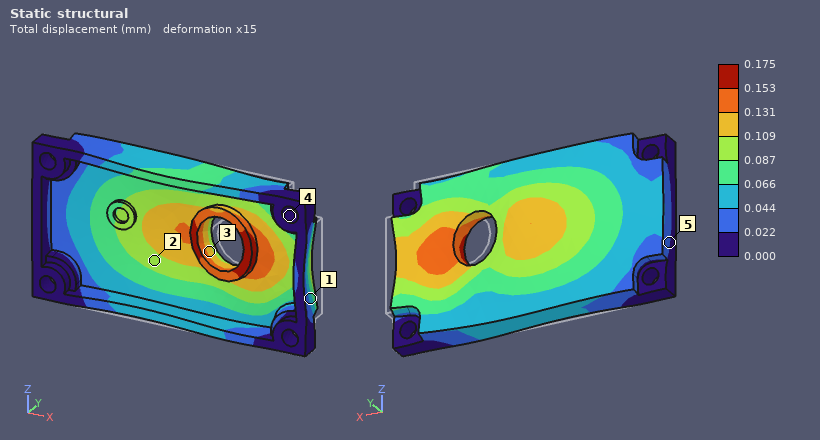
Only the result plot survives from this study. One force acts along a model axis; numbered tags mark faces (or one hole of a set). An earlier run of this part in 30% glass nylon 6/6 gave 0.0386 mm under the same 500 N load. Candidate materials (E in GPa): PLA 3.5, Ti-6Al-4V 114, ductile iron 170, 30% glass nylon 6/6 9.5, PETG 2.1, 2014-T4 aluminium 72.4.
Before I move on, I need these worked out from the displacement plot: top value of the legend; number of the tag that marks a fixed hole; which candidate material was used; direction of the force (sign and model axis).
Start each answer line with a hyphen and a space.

- 0.175 mm
- 4
- PETG
- -X
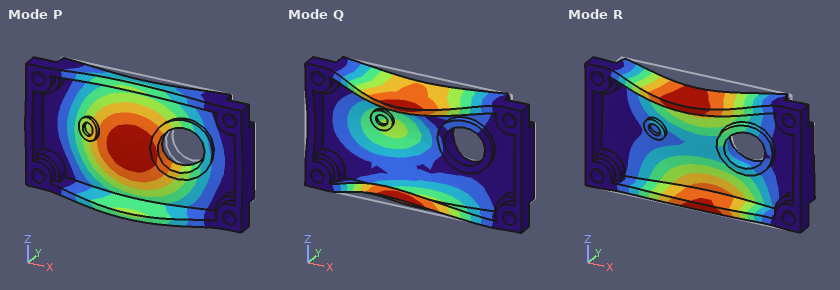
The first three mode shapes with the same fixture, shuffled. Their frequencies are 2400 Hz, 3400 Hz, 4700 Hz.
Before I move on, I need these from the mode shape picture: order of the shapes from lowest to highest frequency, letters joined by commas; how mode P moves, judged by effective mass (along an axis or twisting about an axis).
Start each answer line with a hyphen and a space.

- P, R, Q
- along Y
